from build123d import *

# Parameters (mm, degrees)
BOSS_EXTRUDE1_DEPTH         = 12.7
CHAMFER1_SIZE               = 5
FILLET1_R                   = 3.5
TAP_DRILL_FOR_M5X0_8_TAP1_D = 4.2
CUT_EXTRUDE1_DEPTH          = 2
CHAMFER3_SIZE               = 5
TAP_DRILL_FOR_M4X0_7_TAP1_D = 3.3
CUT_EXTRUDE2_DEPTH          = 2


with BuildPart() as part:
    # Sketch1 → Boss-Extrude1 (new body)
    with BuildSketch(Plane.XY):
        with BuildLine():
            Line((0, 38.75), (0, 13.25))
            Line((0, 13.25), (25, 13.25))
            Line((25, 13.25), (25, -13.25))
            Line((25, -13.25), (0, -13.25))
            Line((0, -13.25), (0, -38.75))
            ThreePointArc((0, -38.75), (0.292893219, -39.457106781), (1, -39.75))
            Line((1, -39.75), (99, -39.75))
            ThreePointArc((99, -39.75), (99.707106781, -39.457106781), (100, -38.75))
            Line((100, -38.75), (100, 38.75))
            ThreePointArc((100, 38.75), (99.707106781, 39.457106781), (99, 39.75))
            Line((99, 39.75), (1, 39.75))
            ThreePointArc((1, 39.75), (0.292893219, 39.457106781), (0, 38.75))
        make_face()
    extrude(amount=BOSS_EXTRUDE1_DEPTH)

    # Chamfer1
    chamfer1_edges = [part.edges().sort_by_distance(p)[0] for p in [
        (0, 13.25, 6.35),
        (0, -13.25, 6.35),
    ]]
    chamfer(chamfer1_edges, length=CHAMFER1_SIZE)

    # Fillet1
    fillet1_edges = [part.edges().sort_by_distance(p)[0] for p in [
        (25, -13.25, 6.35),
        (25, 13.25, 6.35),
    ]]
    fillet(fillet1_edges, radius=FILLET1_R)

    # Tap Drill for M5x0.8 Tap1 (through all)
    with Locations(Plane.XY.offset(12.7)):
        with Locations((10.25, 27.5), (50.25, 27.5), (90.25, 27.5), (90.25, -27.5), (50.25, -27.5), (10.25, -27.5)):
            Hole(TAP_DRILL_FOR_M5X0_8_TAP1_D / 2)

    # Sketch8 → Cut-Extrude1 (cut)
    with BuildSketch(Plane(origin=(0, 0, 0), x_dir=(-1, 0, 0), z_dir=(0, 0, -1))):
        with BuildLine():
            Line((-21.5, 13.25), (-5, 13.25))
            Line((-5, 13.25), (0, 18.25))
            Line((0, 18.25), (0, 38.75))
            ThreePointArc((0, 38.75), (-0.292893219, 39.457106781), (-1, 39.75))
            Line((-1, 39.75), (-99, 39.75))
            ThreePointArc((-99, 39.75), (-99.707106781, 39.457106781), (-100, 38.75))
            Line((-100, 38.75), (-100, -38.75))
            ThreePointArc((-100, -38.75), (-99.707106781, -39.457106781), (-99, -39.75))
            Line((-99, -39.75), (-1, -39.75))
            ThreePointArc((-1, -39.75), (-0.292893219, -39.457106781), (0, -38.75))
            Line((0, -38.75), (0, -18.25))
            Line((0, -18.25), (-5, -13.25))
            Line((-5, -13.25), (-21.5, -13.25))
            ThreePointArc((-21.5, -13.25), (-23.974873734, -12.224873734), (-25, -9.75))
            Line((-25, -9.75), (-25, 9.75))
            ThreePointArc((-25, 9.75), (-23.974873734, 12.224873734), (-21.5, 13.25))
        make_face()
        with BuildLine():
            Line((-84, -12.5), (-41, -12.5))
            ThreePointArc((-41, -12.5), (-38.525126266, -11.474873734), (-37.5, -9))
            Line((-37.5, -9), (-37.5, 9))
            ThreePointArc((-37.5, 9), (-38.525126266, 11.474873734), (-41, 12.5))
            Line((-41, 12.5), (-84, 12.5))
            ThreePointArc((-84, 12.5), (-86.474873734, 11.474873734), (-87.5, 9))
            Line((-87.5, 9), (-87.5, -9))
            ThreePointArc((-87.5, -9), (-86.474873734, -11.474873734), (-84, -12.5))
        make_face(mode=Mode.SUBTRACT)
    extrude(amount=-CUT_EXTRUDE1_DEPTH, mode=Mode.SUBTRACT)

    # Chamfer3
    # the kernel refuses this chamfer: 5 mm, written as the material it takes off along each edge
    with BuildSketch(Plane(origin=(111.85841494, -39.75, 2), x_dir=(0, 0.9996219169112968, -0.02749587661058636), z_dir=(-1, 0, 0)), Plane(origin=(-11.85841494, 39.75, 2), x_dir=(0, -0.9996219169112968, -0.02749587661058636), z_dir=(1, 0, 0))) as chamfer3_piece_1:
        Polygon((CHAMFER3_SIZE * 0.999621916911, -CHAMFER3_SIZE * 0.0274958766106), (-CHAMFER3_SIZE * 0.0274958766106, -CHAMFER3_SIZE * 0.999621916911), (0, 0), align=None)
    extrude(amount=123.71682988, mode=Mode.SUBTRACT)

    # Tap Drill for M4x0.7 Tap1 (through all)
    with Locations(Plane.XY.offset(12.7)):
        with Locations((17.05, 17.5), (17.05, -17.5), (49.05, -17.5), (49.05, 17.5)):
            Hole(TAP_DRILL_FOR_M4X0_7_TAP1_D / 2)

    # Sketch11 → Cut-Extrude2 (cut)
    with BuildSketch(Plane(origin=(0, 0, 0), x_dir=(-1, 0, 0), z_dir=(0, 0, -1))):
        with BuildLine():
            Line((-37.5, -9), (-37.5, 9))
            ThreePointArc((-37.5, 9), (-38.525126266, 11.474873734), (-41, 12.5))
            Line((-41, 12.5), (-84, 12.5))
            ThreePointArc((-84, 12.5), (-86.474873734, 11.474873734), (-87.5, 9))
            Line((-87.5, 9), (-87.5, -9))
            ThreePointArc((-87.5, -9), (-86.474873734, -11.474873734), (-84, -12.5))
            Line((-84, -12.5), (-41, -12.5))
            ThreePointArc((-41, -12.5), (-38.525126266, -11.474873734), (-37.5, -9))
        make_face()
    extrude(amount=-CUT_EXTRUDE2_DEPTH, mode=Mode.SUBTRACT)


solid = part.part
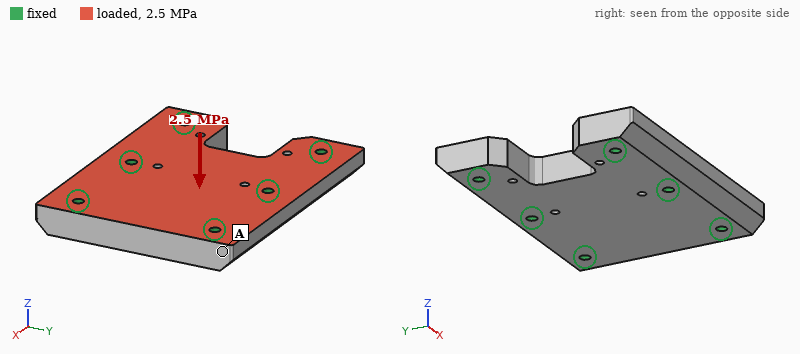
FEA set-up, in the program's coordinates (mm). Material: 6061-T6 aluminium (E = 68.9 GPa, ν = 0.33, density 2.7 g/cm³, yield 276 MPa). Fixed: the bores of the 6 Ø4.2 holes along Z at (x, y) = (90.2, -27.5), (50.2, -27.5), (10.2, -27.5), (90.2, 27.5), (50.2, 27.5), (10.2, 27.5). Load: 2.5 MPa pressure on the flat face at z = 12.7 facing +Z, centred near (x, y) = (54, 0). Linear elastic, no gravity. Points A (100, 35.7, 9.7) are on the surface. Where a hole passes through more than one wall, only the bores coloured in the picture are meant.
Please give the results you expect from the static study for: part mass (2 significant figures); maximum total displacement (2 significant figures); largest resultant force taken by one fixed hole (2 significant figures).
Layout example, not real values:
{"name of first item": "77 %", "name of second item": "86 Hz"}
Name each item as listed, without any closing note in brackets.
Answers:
{"part mass": "200 g", "maximum total displacement": "20 µm", "largest resultant force taken by one fixed hole": "3.9 kN"}
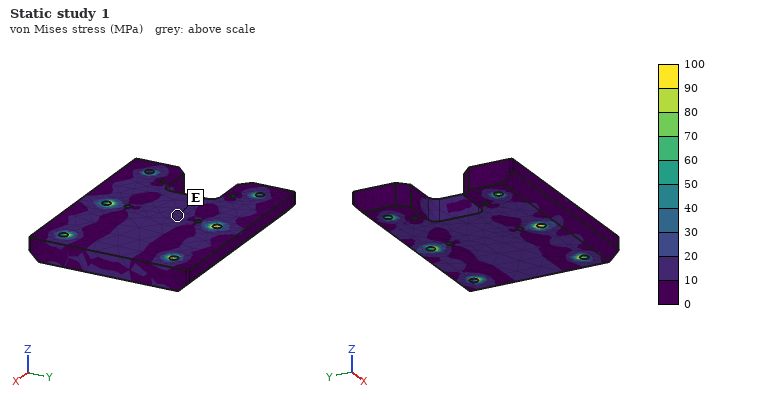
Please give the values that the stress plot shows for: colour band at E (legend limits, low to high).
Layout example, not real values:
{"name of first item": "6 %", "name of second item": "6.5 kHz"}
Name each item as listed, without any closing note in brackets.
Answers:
{"colour band at E": "10 to 20 MPa"}
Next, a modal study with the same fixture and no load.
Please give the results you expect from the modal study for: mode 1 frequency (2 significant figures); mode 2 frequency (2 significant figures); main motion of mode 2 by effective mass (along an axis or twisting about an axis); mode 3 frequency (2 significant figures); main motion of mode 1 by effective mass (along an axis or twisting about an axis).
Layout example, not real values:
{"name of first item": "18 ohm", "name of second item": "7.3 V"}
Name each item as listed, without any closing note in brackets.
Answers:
{"mode 1 frequency": "12 kHz", "mode 2 frequency": "14 kHz", "main motion of mode 2 by effective mass": "twisting about Y", "mode 3 frequency": "19 kHz", "main motion of mode 1 by effective mass": "along Z"}
